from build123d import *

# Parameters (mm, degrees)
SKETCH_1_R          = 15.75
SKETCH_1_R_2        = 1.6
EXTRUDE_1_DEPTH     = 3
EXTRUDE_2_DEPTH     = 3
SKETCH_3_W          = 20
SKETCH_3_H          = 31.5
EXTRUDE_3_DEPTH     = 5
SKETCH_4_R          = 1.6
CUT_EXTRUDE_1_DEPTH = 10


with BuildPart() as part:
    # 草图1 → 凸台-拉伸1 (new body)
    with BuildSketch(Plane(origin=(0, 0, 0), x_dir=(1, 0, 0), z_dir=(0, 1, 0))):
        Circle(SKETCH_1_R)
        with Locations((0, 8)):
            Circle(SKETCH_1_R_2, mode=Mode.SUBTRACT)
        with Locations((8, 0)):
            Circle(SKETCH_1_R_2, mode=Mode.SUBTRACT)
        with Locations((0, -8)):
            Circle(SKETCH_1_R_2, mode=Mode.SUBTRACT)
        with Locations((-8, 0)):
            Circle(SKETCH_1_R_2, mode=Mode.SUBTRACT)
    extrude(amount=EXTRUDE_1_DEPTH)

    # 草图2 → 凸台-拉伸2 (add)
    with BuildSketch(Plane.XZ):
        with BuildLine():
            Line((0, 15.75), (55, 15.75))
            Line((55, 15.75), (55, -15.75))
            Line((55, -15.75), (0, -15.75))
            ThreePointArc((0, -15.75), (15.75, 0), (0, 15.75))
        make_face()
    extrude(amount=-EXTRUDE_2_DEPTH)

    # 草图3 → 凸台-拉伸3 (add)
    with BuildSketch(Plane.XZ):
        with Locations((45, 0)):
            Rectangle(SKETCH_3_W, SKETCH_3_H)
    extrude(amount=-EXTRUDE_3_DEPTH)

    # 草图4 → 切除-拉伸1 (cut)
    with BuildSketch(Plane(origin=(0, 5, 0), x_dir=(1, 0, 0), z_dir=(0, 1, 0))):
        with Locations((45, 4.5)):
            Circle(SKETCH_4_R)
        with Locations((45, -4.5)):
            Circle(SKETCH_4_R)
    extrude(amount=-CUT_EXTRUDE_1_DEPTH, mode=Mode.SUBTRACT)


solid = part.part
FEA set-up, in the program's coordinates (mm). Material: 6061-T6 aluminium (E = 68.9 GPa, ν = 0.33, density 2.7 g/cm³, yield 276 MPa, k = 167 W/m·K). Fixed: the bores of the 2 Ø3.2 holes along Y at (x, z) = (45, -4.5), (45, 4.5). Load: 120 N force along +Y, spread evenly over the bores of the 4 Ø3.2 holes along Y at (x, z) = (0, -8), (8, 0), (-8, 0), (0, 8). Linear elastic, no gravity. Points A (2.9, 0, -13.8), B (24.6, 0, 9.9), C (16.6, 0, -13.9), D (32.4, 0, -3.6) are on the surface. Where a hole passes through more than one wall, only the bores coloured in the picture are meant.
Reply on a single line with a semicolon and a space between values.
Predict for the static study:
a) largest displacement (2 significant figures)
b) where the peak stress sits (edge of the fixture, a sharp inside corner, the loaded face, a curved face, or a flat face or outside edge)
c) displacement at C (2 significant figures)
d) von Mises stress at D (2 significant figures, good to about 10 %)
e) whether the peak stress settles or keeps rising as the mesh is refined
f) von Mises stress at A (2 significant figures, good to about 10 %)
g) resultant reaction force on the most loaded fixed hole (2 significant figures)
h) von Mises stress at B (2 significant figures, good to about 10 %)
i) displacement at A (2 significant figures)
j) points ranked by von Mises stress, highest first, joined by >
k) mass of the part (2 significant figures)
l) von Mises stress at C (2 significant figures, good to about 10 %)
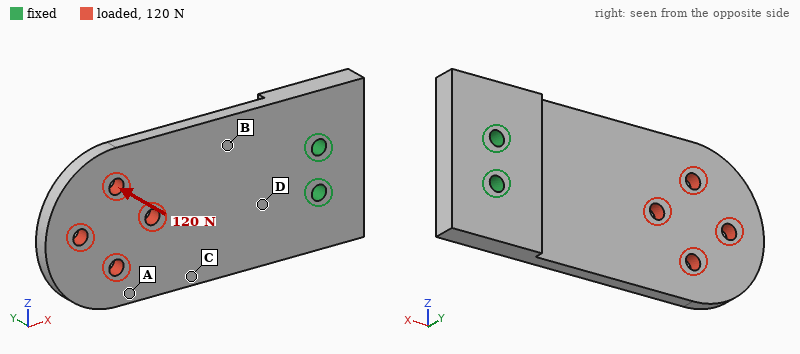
0.74 mm; edge of the fixture; 0.18 mm; 76 MPa; keeps rising; 13 MPa; 60 N; 60 MPa; 0.40 mm; D > B > C > A; 20 g; 43 MPa
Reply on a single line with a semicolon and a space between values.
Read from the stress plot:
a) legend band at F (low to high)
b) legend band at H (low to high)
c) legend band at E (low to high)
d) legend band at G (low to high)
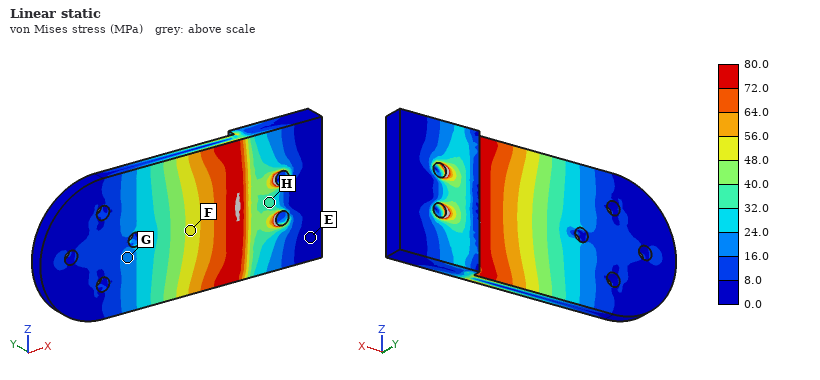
48.0 to 56.0 MPa; 32.0 to 40.0 MPa; 0.0 to 8.0 MPa; 16.0 to 24.0 MPa
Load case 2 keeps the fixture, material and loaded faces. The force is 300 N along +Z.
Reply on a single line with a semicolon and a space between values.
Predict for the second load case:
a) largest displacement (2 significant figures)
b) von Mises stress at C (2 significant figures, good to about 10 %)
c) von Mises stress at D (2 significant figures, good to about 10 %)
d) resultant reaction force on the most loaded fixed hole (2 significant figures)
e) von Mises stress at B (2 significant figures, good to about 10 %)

50 µm; 8.6 MPa; 8.9 MPa; 1.2 kN; 9.3 MPa
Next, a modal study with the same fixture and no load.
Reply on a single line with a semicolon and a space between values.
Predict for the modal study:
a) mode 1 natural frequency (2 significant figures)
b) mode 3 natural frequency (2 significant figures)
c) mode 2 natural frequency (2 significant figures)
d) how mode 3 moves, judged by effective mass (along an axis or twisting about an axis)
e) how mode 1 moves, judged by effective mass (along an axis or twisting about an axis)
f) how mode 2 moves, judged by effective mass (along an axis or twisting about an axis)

960 Hz; 5200 Hz; 3400 Hz; along Z; along Y; twisting about X
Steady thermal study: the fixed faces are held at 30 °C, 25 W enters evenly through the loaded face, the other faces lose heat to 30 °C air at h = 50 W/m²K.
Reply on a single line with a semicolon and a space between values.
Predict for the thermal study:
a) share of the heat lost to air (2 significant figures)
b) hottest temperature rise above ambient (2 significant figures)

25 %; 58 K
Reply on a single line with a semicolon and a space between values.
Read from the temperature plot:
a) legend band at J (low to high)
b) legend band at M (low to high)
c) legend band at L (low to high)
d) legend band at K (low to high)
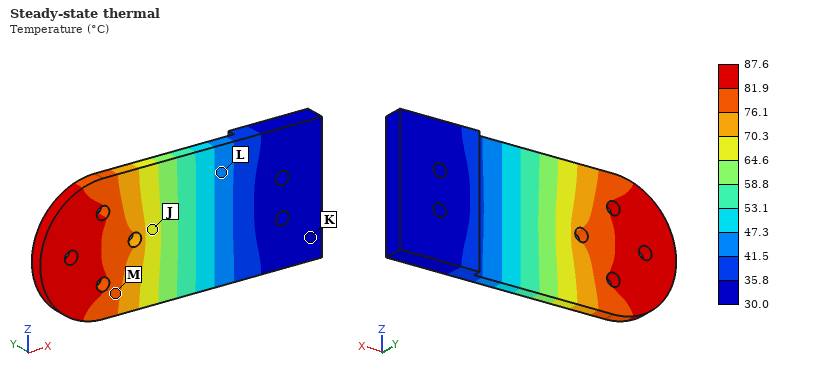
64.6 to 70.3 °C; 76.1 to 81.9 °C; 41.5 to 47.3 °C; 30.0 to 35.8 °C
